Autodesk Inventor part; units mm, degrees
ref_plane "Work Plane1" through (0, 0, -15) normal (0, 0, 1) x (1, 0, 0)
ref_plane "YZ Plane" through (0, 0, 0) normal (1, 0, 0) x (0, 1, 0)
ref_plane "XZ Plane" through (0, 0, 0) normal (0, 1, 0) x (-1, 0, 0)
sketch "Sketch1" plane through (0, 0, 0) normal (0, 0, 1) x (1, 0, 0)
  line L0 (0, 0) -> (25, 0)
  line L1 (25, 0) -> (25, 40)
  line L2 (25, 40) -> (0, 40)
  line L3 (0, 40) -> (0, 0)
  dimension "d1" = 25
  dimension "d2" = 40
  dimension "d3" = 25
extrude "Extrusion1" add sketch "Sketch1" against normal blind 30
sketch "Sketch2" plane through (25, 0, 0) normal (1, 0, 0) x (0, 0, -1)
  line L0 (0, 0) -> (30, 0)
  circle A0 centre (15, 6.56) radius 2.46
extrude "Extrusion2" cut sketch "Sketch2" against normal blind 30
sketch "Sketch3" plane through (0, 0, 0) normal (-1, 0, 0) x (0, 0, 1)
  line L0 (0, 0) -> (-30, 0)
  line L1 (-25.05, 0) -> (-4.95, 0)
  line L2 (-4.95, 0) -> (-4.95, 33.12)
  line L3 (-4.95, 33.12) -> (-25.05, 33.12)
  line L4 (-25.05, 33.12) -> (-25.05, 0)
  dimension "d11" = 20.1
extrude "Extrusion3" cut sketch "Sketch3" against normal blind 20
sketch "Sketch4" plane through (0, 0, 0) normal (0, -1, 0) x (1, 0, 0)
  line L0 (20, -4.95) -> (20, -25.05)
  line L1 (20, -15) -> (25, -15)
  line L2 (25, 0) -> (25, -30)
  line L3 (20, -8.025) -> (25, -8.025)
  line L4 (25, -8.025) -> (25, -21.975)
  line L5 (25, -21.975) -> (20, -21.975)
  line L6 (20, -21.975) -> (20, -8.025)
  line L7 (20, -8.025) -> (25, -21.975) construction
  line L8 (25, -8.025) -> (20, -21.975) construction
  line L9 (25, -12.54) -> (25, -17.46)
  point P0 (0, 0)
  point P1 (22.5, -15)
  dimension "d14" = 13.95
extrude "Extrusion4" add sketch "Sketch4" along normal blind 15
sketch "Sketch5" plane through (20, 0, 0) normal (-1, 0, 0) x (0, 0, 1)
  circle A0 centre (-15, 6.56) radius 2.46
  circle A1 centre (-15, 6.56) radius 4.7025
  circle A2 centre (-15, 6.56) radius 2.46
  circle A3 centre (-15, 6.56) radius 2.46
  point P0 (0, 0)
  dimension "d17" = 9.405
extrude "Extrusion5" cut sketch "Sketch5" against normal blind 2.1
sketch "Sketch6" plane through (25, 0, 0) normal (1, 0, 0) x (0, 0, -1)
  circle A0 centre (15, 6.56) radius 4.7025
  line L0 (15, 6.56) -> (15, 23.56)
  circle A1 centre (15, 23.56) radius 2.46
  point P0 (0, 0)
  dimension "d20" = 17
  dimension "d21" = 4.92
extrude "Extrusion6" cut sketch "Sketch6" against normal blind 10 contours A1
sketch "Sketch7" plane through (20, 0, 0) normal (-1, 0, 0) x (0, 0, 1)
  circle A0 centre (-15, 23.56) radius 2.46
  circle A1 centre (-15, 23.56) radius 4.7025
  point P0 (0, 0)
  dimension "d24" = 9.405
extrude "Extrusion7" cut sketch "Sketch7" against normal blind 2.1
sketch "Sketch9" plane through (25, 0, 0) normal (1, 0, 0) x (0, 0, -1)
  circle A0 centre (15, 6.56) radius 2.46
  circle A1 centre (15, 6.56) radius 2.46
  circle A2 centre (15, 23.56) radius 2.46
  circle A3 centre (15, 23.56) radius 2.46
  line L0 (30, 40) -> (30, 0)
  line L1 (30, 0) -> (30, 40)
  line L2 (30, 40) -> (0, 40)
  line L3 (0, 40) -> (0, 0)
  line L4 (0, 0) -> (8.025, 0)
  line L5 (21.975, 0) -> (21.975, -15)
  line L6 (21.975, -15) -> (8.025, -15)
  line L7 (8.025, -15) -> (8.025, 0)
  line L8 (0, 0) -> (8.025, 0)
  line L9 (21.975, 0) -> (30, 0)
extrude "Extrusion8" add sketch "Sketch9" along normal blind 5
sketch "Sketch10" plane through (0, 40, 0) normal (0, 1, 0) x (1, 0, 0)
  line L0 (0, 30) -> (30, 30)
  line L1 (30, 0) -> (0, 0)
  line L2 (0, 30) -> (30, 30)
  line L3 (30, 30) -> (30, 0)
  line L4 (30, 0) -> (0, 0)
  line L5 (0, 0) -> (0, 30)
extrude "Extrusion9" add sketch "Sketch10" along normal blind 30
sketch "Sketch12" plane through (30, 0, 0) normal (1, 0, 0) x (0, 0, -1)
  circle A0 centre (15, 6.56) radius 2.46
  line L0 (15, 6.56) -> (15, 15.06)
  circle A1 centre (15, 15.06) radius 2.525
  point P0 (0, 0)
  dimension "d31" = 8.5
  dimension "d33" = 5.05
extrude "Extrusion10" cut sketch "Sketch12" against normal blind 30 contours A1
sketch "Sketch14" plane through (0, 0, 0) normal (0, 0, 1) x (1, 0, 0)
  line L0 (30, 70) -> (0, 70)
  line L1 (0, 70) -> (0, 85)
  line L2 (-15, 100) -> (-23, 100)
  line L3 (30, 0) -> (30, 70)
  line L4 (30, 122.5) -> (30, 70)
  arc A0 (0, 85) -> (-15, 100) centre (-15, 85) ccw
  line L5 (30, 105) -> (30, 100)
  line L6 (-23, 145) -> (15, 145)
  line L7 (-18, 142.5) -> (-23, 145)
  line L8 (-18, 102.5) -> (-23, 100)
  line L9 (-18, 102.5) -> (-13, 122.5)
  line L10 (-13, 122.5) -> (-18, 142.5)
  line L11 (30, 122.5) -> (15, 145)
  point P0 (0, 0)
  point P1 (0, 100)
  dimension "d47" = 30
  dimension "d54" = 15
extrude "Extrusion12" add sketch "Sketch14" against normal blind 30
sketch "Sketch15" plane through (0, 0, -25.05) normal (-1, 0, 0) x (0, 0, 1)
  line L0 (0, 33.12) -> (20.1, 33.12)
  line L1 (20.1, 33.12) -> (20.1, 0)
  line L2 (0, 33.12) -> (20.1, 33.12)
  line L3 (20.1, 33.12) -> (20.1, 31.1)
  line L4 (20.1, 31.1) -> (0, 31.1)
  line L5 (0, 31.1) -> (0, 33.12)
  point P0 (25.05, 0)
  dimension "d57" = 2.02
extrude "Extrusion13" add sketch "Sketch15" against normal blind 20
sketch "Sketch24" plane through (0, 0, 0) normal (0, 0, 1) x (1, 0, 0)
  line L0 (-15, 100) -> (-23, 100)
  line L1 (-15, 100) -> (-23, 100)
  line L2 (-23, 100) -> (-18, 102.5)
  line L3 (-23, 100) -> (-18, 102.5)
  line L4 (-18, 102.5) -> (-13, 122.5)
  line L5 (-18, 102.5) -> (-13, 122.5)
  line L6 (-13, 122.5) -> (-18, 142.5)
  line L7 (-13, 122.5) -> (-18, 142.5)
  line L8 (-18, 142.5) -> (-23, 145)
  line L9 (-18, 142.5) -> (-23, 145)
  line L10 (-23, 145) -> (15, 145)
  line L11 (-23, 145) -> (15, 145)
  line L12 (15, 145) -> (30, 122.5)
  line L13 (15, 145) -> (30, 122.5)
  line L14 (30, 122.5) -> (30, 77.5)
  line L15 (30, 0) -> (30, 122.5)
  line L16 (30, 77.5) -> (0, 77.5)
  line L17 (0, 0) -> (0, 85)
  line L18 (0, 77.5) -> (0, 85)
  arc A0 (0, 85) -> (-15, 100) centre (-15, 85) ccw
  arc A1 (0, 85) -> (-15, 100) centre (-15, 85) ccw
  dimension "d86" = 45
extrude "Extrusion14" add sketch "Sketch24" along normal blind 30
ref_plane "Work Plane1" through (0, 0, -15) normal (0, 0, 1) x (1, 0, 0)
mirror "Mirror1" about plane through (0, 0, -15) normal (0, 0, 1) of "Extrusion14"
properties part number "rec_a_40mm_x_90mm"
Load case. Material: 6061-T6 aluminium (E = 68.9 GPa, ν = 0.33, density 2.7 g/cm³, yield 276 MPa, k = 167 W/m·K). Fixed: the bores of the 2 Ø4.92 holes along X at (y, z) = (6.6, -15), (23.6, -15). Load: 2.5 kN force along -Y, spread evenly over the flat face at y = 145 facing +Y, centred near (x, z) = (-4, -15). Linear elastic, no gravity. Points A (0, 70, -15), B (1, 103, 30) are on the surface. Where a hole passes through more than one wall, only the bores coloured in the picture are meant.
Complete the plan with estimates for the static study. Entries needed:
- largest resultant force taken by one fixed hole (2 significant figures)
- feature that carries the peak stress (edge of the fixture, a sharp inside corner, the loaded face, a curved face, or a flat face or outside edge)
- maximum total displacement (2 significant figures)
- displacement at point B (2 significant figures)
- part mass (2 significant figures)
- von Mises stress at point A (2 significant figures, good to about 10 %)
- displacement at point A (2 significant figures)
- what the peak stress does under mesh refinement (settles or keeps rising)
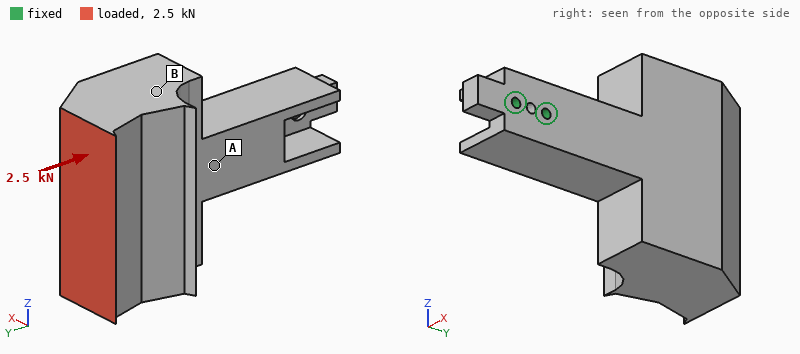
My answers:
3.4 kN
edge of the fixture
0.27 mm
0.16 mm
800 g
12 MPa
0.098 mm
keeps rising
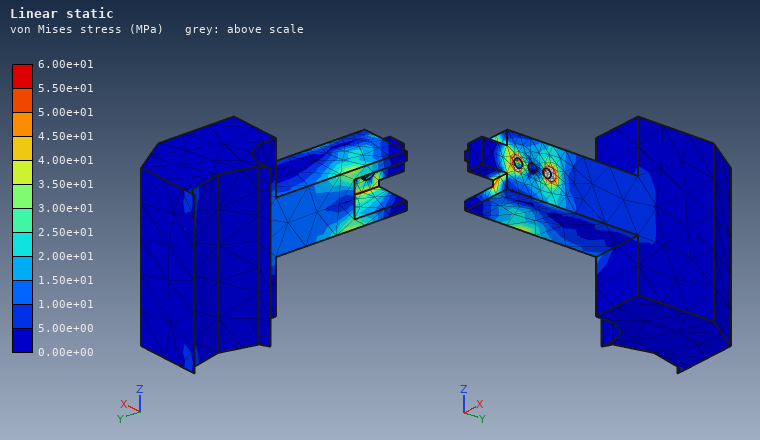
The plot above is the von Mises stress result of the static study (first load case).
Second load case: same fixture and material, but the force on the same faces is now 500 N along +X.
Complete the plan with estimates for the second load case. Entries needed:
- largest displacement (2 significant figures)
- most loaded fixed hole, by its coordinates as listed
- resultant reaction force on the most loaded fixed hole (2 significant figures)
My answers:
0.23 mm
(23.6, -15)
2.9 kN
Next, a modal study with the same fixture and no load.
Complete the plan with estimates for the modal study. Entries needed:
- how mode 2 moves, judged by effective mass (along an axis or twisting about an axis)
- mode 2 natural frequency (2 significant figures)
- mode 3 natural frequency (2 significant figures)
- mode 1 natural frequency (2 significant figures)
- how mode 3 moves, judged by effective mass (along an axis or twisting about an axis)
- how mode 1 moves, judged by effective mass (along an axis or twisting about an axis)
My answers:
along Z
450 Hz
850 Hz
400 Hz
twisting about Y
along X
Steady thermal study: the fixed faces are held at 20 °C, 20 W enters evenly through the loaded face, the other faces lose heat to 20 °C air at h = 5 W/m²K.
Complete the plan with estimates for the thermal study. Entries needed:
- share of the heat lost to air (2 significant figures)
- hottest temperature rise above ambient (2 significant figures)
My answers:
8.0 %
14 K
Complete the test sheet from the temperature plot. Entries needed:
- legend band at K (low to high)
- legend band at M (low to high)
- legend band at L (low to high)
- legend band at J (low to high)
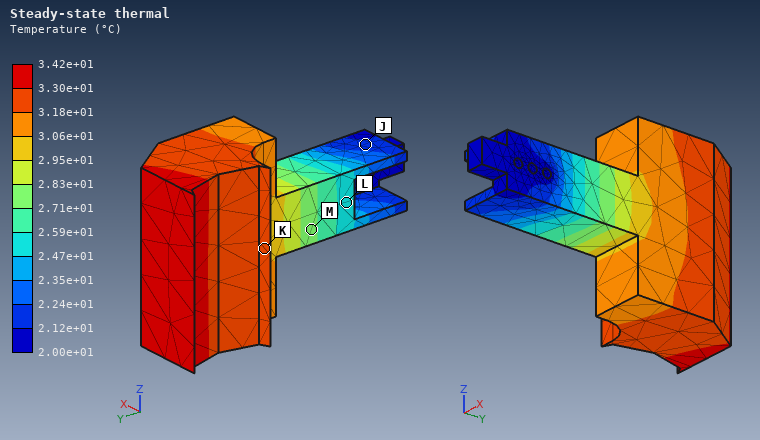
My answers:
3.18e+01 to 3.30e+01 °C
2.71e+01 to 2.83e+01 °C
2.47e+01 to 2.59e+01 °C
2.12e+01 to 2.24e+01 °C
